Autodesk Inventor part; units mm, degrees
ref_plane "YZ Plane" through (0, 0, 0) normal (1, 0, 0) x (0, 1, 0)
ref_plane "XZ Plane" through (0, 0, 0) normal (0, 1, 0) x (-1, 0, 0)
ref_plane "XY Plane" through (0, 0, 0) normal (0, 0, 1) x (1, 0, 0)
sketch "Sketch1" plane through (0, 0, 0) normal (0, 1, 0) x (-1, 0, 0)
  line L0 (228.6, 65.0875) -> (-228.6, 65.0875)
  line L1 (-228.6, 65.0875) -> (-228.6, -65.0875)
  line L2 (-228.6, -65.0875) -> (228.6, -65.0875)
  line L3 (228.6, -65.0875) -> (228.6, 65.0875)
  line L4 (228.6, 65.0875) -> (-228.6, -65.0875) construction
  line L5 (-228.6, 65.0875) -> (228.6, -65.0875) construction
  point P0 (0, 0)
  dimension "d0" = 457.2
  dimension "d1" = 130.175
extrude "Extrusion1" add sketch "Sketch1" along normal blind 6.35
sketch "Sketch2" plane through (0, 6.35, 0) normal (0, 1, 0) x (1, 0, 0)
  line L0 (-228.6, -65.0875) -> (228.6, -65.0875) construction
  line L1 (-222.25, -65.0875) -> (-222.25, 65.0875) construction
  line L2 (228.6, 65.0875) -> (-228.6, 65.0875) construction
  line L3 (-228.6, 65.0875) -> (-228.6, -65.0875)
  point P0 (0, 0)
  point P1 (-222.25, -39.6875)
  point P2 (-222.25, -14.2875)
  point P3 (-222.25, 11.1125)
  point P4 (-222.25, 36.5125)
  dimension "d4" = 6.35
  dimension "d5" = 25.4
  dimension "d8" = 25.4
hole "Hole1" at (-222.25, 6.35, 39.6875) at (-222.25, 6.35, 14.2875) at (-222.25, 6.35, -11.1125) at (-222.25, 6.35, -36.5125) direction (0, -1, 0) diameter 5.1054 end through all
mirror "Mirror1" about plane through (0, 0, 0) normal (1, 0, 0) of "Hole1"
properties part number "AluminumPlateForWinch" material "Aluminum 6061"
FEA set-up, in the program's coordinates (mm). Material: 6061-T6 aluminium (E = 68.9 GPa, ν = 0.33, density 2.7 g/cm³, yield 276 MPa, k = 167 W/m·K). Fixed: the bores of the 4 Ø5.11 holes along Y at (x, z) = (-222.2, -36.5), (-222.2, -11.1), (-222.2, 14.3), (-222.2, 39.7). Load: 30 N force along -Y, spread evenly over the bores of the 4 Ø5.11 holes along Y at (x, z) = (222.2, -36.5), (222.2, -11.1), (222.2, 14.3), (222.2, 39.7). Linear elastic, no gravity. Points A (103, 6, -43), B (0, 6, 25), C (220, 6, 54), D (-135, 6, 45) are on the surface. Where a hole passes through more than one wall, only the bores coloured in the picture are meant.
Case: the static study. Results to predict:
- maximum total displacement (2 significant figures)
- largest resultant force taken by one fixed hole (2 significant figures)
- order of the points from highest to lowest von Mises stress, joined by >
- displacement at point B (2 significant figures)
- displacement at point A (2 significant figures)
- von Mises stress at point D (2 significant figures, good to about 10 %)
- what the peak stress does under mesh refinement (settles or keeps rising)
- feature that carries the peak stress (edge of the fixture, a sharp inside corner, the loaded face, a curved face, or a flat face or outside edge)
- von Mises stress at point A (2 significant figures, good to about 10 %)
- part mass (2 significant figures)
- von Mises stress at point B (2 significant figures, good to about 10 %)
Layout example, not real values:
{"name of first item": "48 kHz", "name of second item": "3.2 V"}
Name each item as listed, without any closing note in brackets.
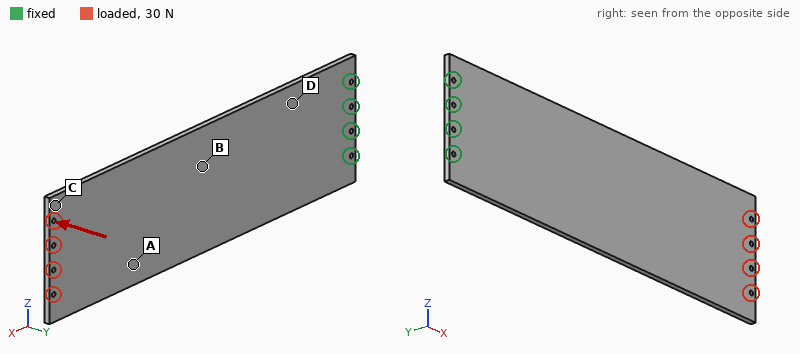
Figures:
{"maximum total displacement": "4.7 mm", "largest resultant force taken by one fixed hole": "49 N", "order of the points from highest to lowest von Mises stress, joined by >": "D > B > A > C", "displacement at point B": "1.4 mm", "displacement at point A": "2.8 mm", "von Mises stress at point D": "12 MPa", "what the peak stress does under mesh refinement": "keeps rising", "feature that carries the peak stress": "edge of the fixture", "von Mises stress at point A": "4.1 MPa", "part mass": "1.0 kg", "von Mises stress at point B": "7.6 MPa"}
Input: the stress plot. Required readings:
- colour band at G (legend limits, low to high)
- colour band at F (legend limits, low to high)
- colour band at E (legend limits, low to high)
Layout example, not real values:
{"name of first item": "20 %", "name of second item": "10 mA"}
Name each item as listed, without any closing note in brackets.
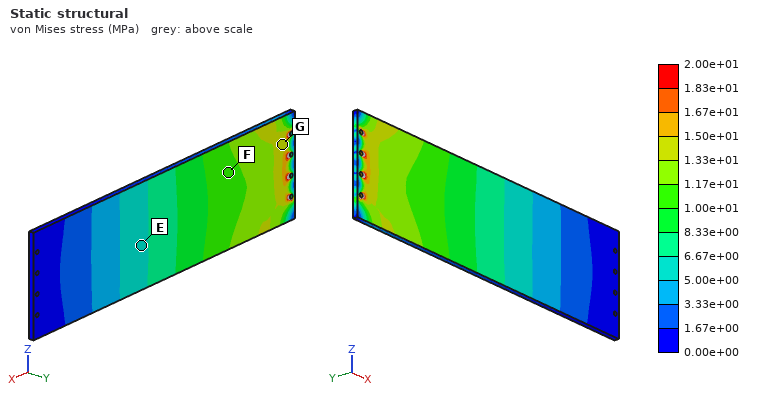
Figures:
{"colour band at G": "1.33e+01 to 1.50e+01 MPa", "colour band at F": "1.00e+01 to 1.17e+01 MPa", "colour band at E": "5.00e+00 to 6.67e+00 MPa"}
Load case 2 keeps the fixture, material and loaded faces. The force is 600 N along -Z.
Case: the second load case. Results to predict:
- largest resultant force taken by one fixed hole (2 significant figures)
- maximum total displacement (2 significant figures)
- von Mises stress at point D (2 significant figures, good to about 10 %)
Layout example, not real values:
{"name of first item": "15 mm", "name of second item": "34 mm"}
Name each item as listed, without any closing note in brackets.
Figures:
{"largest resultant force taken by one fixed hole": "3.1 kN", "maximum total displacement": "0.31 mm", "von Mises stress at point D": "8.4 MPa"}
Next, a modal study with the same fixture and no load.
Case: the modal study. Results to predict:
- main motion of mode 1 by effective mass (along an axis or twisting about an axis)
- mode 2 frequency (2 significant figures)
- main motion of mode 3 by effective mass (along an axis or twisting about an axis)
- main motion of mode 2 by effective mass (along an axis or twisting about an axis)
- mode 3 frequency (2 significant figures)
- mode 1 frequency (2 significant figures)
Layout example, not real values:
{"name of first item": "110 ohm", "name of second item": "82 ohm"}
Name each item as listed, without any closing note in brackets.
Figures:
{"main motion of mode 1 by effective mass": "along Y", "mode 2 frequency": "160 Hz", "main motion of mode 3 by effective mass": "twisting about X", "main motion of mode 2 by effective mass": "along Y", "mode 3 frequency": "180 Hz", "mode 1 frequency": "26 Hz"}
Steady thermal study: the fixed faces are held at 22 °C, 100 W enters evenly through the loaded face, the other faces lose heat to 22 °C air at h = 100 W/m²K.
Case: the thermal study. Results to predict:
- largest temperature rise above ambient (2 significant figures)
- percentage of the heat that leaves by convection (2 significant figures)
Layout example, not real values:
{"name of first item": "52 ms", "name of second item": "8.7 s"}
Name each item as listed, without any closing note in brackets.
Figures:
{"largest temperature rise above ambient": "55 K", "percentage of the heat that leaves by convection": "100 %"}
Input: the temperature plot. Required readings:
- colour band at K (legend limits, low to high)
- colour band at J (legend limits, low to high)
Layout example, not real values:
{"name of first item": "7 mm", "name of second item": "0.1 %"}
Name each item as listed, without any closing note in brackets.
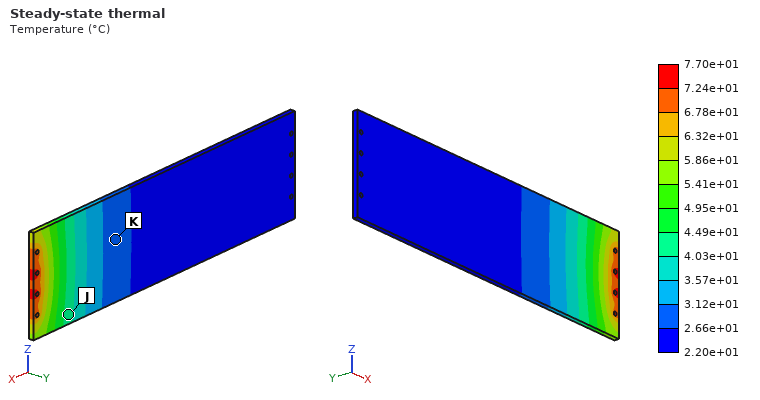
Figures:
{"colour band at K": "2.66e+01 to 3.12e+01 °C", "colour band at J": "4.03e+01 to 4.49e+01 °C"}
